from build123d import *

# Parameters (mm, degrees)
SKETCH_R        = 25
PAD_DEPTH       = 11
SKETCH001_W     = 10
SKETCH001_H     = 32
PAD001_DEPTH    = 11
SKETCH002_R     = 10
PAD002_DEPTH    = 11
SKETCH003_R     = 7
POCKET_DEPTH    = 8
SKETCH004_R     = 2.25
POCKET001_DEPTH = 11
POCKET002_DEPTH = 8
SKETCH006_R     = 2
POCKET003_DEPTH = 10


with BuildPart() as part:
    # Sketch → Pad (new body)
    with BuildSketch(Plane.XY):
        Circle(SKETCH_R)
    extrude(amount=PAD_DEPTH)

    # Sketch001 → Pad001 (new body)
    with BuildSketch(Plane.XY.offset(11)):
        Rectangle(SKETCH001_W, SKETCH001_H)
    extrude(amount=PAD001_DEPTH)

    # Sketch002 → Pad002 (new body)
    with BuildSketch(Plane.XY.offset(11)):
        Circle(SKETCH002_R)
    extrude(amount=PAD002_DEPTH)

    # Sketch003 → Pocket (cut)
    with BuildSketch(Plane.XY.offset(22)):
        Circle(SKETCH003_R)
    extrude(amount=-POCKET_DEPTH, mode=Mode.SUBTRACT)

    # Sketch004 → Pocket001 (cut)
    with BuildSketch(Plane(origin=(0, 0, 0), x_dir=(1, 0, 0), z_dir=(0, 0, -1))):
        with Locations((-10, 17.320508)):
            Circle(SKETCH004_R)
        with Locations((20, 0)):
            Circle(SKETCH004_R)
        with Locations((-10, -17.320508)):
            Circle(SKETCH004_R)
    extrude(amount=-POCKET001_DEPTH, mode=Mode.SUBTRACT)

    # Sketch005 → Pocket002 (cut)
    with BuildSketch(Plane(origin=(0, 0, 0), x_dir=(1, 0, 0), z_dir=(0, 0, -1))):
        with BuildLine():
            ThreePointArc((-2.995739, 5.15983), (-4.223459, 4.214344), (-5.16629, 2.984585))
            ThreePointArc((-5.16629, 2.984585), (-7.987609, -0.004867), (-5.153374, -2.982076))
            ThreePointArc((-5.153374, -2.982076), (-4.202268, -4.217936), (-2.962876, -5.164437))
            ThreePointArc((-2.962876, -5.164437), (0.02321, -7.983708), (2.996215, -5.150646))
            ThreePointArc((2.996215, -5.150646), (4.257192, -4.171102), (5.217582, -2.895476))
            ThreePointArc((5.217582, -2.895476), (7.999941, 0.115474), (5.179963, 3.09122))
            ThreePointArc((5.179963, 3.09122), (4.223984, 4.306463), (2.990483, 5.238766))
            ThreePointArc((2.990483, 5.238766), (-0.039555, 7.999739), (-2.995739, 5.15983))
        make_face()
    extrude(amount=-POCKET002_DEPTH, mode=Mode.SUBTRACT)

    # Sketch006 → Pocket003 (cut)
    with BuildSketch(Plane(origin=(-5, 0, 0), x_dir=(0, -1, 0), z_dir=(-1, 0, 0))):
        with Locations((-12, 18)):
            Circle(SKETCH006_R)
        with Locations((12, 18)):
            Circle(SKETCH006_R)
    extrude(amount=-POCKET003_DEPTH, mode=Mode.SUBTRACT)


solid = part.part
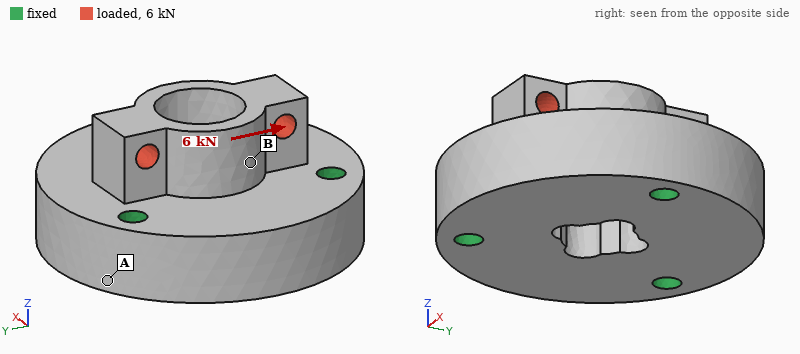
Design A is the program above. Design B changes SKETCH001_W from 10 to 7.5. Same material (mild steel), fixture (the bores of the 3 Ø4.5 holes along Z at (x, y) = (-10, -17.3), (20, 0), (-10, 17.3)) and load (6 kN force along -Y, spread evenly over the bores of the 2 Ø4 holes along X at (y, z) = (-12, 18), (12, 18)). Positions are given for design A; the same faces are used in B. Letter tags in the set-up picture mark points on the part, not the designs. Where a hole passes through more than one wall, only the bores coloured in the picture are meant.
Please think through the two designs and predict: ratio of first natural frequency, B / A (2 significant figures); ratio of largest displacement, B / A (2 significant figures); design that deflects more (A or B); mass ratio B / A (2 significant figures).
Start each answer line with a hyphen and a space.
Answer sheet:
- 1.0
- 1.2
- B
- 0.99
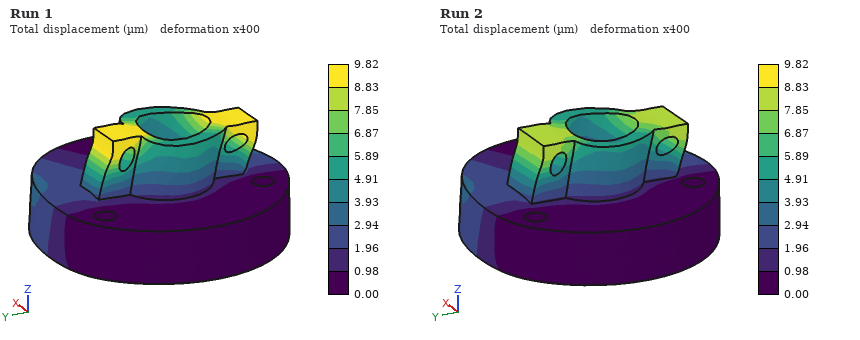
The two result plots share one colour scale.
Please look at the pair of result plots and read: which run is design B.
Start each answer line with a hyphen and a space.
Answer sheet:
- Run 1
